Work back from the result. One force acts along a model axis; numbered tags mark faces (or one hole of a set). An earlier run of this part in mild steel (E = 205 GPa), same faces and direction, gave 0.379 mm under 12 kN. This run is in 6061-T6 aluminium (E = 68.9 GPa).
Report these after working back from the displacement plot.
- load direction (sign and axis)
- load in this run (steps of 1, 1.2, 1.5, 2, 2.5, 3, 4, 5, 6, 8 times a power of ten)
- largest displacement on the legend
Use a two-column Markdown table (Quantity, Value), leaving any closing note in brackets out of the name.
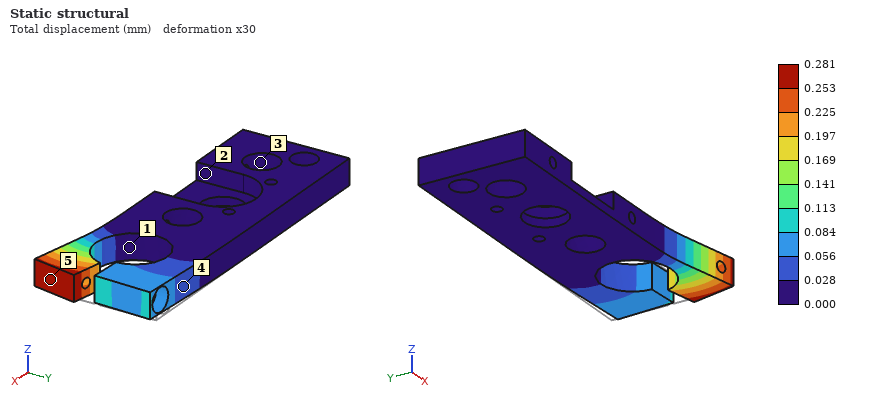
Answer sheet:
| Quantity | Value |
|---|---|
| load direction | -Y |
| load in this run | 3 kN |
| largest displacement on the legend | 0.281 mm |
